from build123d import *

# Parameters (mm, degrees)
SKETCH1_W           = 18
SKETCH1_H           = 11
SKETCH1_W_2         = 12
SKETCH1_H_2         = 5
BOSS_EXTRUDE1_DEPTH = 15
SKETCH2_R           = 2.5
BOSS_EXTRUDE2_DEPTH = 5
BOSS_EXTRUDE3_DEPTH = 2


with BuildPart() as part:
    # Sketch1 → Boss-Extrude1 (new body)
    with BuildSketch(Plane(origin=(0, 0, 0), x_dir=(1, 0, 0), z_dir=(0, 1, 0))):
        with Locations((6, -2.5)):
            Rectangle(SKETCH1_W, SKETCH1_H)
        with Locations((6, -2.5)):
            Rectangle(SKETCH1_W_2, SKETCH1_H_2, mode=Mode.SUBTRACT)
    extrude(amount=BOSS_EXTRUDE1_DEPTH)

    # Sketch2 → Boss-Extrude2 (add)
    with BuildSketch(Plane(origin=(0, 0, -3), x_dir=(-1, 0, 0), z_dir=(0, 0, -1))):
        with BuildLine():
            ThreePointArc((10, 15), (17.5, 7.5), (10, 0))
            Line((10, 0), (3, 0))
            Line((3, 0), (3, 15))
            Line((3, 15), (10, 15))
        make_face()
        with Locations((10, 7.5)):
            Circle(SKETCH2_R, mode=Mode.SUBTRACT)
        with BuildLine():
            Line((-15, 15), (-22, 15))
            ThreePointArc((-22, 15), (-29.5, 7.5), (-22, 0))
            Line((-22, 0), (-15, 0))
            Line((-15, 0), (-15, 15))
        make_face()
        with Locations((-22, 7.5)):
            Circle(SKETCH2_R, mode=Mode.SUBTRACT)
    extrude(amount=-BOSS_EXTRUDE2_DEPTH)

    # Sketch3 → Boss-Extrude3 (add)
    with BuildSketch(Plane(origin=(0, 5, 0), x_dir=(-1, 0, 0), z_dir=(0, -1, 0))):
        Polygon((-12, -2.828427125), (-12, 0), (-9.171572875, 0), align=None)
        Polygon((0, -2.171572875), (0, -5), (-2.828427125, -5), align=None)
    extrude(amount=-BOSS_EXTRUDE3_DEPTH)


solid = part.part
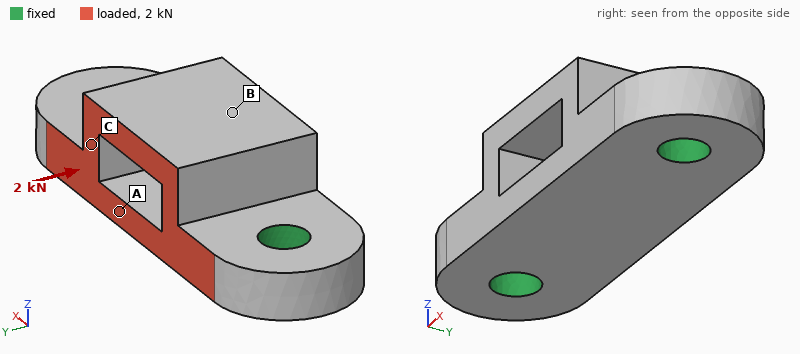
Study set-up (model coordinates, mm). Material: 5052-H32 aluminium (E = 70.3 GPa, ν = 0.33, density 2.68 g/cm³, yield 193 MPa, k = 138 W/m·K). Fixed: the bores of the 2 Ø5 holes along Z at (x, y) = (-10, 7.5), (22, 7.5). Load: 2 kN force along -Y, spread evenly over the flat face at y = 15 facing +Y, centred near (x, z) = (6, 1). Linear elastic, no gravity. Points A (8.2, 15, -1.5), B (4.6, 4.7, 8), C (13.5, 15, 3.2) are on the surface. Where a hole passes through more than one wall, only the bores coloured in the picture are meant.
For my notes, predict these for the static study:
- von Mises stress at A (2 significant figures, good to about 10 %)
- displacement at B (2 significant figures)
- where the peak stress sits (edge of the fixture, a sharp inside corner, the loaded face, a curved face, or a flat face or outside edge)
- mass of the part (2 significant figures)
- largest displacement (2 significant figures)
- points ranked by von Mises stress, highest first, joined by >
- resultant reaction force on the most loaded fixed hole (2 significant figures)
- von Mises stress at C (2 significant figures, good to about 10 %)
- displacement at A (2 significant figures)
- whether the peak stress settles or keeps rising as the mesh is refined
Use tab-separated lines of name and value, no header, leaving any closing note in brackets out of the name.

von Mises stress at A	28 MPa
displacement at B	15 µm
where the peak stress sits	edge of the fixture
mass of the part	10 g
largest displacement	18 µm
points ranked by von Mises stress, highest first, joined by >	A > C > B
resultant reaction force on the most loaded fixed hole	1.0 kN
von Mises stress at C	17 MPa
displacement at A	9.2 µm
whether the peak stress settles or keeps rising as the mesh is refined	keeps rising
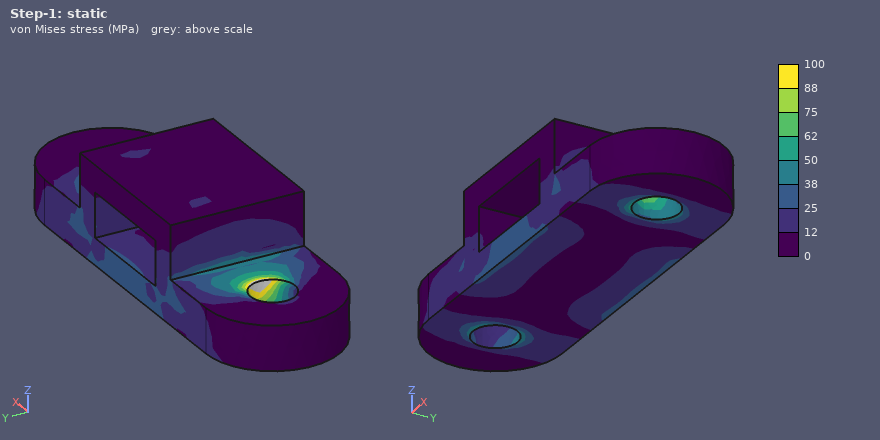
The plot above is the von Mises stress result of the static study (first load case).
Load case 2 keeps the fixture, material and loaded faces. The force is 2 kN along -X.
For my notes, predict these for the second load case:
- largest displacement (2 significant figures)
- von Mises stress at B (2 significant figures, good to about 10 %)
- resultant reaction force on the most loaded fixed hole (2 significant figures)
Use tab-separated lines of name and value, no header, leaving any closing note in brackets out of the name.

largest displacement	14 µm
von Mises stress at B	8.4 MPa
resultant reaction force on the most loaded fixed hole	1.1 kN
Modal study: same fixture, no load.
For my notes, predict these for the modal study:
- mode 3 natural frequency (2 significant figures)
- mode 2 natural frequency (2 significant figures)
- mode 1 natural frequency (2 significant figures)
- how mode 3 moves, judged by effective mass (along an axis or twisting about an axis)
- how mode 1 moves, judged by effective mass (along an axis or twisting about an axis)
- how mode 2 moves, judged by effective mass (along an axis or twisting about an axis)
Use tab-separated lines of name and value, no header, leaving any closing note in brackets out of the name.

mode 3 natural frequency	34 kHz
mode 2 natural frequency	26 kHz
mode 1 natural frequency	20 kHz
how mode 3 moves, judged by effective mass	along X
how mode 1 moves, judged by effective mass	along Y
how mode 2 moves, judged by effective mass	along Z
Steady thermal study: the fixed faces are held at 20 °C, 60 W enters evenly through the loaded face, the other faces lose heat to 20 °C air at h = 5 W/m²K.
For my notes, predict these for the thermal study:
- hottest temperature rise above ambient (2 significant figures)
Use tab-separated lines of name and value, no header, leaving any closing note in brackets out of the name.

hottest temperature rise above ambient	38 K
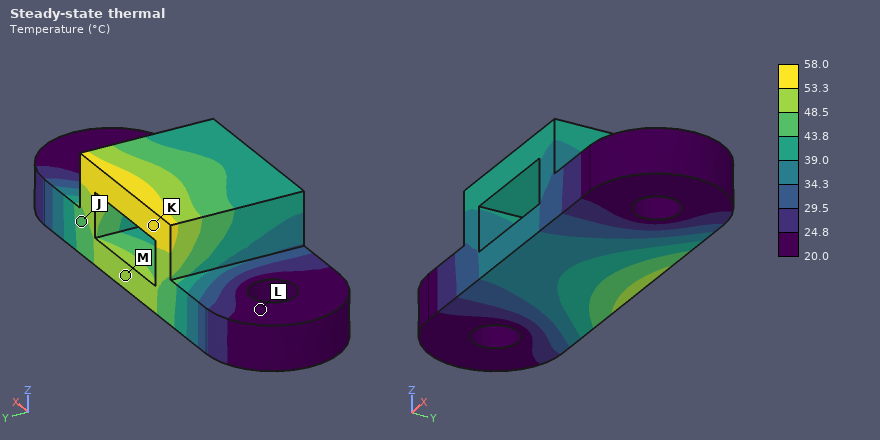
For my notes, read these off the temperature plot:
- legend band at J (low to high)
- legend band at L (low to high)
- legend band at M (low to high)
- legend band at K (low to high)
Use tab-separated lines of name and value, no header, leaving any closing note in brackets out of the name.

legend band at J	43.8 to 48.5 °C
legend band at L	20.0 to 24.8 °C
legend band at M	48.5 to 53.3 °C
legend band at K	53.3 to 58.0 °C
